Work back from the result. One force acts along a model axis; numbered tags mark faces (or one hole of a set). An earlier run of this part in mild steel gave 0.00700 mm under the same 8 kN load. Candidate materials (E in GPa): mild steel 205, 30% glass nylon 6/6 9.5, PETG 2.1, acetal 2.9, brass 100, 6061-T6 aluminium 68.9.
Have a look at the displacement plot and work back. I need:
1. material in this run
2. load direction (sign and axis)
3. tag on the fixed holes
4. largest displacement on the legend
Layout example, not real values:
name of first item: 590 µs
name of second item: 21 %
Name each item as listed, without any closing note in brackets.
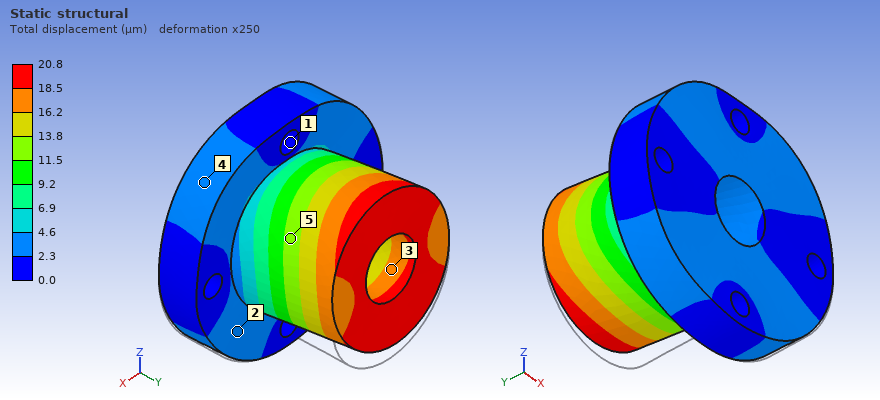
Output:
material in this run: 6061-T6 aluminium
load direction: +Z
tag on the fixed holes: 1
largest displacement on the legend: 20.8 µm
